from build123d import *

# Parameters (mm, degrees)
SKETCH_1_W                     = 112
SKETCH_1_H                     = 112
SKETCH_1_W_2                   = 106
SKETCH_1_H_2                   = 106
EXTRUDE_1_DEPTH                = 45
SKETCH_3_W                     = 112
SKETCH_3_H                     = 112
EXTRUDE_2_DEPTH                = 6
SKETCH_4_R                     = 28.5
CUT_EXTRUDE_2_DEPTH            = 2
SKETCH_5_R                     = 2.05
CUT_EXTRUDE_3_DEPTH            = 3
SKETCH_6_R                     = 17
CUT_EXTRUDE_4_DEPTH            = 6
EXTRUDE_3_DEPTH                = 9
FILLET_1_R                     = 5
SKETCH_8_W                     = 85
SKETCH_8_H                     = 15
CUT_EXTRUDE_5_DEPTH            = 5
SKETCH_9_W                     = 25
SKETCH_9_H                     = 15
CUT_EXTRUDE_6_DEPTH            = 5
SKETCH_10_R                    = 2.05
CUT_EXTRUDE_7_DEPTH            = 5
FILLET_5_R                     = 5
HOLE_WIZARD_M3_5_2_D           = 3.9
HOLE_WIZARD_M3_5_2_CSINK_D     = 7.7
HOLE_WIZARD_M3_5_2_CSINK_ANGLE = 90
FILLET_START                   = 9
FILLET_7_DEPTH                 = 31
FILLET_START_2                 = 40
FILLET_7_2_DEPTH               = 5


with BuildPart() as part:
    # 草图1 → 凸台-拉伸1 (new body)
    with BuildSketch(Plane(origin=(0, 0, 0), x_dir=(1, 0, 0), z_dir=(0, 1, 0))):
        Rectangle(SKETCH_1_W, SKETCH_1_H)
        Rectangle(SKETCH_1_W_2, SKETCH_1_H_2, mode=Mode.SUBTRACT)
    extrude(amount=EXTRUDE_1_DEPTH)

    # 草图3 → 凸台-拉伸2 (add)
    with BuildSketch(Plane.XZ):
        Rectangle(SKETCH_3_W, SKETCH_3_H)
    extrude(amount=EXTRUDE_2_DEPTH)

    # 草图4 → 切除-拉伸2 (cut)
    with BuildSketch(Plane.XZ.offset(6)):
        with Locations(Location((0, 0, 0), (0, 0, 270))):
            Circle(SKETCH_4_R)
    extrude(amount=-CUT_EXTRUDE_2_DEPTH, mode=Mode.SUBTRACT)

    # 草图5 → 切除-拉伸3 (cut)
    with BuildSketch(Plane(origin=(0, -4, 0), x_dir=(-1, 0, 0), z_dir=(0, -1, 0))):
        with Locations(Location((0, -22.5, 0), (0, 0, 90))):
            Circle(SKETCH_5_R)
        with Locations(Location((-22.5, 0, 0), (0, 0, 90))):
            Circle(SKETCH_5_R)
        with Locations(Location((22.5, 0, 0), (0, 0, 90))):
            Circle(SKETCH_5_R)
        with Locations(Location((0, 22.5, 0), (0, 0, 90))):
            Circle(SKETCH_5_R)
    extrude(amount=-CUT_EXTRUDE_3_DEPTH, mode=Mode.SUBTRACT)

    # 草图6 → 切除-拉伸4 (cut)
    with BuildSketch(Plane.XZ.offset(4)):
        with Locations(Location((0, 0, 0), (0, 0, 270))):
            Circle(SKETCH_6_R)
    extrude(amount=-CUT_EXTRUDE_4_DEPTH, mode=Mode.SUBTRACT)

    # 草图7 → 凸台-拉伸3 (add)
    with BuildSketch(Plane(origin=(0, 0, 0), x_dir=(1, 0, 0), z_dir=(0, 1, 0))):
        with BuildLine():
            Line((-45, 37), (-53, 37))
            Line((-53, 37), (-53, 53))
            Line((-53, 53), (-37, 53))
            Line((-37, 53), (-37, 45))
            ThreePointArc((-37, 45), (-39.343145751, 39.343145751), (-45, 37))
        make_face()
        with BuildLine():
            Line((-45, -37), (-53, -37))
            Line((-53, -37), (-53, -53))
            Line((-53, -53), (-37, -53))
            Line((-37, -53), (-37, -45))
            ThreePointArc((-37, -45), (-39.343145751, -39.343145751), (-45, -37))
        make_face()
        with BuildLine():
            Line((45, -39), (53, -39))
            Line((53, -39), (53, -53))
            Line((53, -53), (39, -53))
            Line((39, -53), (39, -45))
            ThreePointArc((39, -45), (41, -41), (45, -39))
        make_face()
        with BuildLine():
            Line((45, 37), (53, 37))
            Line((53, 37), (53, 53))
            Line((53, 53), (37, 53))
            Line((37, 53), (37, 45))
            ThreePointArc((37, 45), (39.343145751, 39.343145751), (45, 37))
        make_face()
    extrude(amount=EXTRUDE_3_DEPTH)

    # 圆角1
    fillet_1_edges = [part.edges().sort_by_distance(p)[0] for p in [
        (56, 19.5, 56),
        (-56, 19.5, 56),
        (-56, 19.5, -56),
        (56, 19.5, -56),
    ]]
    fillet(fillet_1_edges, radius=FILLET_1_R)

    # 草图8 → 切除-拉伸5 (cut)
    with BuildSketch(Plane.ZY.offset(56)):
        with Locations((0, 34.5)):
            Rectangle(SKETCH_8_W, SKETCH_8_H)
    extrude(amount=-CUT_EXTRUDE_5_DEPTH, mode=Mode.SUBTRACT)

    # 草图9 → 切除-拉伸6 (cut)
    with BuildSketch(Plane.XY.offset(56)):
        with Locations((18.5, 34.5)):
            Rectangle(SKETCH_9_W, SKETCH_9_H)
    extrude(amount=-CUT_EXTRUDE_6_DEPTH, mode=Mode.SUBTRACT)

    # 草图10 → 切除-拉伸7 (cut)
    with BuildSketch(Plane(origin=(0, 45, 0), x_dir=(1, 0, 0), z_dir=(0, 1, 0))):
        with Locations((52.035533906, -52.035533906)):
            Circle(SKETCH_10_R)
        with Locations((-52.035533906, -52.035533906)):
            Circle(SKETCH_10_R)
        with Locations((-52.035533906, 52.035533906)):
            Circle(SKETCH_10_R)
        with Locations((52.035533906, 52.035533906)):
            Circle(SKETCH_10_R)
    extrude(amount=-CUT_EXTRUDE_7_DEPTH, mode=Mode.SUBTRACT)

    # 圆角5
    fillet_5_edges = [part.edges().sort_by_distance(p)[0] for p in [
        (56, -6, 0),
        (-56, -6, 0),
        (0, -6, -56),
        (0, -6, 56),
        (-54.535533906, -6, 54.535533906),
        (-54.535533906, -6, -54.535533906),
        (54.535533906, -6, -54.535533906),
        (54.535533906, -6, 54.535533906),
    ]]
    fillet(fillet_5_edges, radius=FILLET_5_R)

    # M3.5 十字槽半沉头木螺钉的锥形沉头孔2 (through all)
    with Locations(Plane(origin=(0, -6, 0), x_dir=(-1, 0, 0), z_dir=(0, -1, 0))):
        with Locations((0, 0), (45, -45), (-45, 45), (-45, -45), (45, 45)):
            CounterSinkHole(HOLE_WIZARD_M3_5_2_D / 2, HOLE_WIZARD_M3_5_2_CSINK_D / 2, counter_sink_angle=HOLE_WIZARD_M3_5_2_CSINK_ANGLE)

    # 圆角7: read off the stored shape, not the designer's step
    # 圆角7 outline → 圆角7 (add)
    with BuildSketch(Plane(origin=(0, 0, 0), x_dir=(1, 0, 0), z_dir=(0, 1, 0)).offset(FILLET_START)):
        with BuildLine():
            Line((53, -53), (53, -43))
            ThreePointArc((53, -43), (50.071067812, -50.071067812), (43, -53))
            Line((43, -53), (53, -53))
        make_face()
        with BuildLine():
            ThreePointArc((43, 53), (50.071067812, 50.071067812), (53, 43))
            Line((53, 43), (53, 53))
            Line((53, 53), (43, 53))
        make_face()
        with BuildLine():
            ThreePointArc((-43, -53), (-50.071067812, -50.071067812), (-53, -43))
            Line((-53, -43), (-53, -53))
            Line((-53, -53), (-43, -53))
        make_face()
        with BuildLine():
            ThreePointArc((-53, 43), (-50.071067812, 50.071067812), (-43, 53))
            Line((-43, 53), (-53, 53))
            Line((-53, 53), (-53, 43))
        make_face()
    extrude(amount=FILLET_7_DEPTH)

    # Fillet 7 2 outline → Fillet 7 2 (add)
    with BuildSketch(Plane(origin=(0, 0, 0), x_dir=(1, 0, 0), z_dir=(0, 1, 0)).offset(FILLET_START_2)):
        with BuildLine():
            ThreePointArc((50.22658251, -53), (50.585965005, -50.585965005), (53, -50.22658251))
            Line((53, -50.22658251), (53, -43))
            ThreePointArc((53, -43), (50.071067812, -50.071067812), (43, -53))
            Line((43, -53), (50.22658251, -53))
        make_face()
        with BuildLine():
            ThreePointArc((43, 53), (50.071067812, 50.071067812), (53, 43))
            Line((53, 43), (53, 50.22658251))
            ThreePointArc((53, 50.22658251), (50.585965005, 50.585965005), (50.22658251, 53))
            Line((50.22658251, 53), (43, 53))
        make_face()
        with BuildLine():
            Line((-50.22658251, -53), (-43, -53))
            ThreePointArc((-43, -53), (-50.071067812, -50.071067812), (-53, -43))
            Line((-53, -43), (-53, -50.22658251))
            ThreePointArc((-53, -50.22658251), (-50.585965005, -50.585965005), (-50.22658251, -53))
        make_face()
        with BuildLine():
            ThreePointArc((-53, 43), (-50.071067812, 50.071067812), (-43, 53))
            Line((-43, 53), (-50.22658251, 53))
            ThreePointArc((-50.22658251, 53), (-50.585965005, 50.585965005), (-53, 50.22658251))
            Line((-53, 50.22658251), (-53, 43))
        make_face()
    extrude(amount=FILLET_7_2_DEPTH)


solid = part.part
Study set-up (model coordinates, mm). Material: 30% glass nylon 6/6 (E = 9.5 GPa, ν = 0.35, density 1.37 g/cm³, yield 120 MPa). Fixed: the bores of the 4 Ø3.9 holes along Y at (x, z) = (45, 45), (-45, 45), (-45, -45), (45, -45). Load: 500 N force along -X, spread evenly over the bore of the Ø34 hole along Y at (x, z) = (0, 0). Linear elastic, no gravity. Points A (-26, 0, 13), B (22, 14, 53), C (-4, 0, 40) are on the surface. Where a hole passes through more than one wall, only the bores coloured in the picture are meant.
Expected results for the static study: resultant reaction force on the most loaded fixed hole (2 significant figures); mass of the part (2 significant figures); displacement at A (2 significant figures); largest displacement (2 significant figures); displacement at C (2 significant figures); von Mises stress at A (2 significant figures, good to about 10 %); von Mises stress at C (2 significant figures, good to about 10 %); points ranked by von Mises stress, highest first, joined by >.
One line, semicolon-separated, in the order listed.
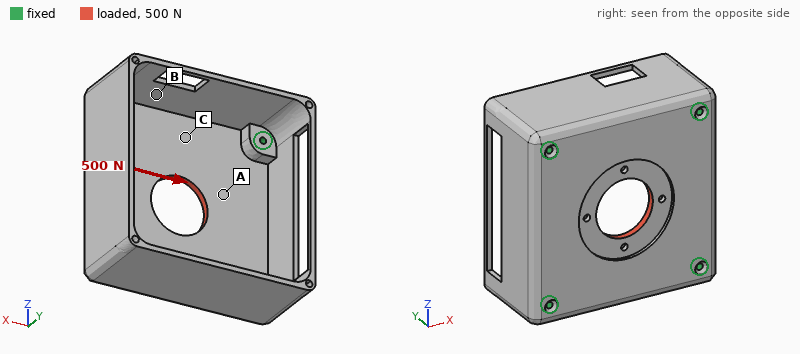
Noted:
140 N; 170 g; 5.7 µm; 8.1 µm; 2.3 µm; 1.0 MPa; 0.55 MPa; A > C > B
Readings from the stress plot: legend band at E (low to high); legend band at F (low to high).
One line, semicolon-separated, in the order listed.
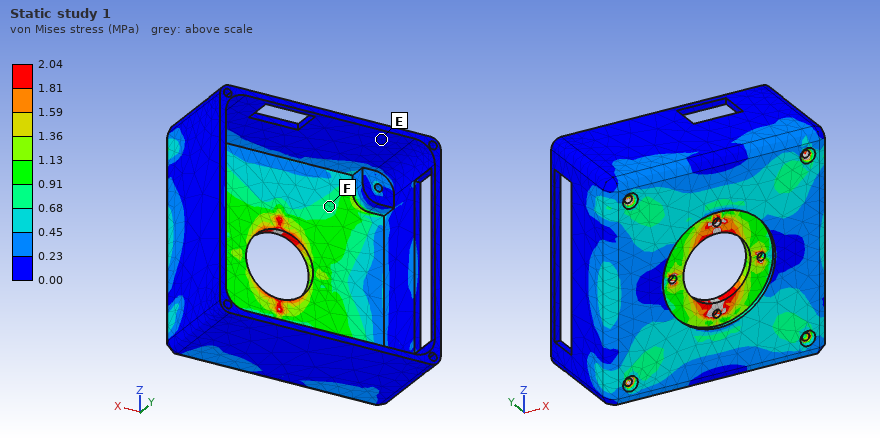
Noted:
0.00 to 0.23 MPa; 0.68 to 0.91 MPa
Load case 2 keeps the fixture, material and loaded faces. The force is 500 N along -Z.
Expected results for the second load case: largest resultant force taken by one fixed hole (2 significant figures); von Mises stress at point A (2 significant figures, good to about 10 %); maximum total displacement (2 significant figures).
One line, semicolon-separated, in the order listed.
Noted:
140 N; 0.85 MPa; 8.1 µm
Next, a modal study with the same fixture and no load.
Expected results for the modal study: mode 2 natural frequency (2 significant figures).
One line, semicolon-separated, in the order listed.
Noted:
1000 Hz
